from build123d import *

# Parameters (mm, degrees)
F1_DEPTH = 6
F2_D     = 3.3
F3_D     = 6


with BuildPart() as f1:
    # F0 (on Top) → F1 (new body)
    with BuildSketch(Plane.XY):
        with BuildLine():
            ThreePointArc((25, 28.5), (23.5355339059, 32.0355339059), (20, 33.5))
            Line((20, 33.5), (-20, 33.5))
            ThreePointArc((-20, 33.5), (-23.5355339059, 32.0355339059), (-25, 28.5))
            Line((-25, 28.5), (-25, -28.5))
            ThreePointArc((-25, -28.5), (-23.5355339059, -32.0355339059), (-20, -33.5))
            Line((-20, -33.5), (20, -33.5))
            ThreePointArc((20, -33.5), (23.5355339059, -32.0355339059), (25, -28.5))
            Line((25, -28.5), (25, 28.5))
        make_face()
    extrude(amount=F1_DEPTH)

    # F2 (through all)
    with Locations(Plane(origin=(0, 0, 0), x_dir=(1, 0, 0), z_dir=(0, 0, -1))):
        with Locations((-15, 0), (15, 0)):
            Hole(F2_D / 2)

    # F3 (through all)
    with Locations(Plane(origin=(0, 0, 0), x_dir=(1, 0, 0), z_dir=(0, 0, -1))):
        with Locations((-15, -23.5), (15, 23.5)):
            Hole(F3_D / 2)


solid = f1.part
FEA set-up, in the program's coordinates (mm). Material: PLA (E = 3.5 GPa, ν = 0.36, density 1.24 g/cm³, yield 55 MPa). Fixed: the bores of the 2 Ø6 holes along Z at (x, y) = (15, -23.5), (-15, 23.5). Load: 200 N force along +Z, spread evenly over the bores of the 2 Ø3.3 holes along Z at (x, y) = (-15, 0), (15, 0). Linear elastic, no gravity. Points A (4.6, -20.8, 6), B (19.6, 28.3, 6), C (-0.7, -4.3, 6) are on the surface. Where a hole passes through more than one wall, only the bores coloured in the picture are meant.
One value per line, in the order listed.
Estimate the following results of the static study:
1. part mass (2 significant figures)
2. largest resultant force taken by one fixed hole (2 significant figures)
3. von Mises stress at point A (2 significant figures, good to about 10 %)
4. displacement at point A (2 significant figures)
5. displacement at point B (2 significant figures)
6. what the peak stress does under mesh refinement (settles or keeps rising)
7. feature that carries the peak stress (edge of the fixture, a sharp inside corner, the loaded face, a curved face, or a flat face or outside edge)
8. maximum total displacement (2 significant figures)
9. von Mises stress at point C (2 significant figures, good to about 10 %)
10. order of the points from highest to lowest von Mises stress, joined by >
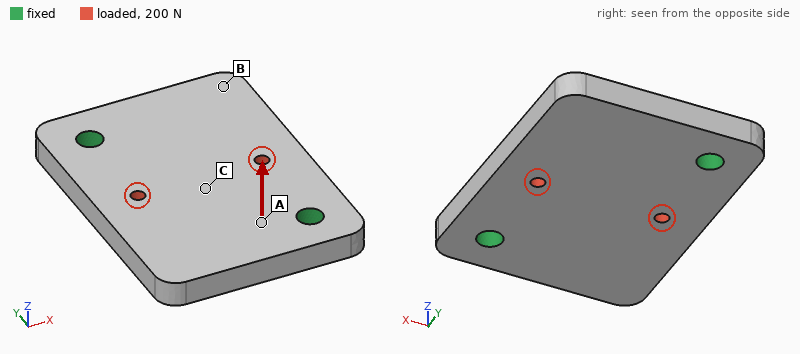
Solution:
24 g
100 N
2.2 MPa
0.022 mm
0.079 mm
keeps rising
edge of the fixture
0.12 mm
3.5 MPa
C > A > B
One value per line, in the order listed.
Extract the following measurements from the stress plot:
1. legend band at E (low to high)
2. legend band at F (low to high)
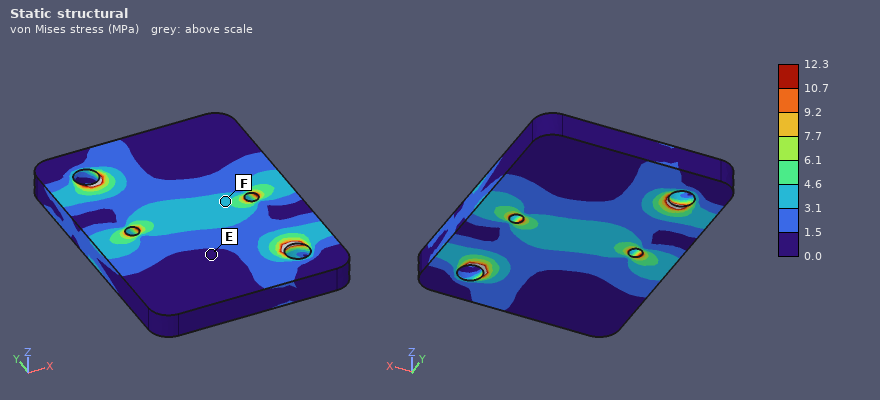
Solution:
0.0 to 1.5 MPa
3.1 to 4.6 MPa
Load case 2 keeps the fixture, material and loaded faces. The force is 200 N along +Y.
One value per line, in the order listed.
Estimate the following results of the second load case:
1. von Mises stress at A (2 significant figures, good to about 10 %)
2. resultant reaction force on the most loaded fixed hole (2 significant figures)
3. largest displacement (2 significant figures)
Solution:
0.26 MPa
100 N
7.9 µm
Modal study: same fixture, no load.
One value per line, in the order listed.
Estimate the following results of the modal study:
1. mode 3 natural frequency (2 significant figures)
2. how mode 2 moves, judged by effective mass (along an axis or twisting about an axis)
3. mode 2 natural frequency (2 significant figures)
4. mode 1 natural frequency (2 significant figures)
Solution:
3400 Hz
along Z
1700 Hz
1300 Hz
